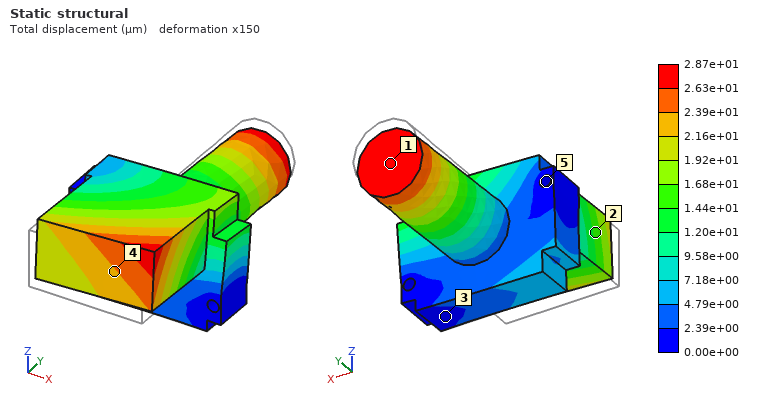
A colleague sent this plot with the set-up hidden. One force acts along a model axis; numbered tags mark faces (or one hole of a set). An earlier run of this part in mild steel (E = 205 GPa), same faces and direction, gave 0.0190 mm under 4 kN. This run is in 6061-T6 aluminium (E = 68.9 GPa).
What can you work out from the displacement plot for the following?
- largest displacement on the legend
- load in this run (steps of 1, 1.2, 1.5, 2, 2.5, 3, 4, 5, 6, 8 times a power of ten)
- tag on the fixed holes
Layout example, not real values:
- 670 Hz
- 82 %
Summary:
- 2.87e+01 µm
- 2 kN
- 5
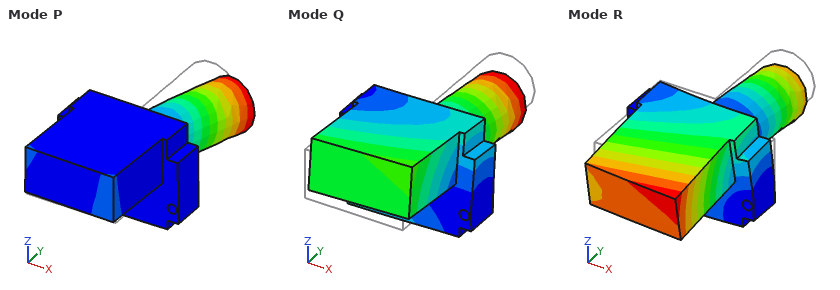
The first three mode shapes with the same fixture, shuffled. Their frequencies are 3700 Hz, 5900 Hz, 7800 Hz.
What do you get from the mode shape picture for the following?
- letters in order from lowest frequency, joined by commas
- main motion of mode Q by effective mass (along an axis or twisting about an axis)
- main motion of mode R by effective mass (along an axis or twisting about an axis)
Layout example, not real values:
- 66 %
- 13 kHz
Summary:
- Q, P, R
- twisting about X
- along Z
